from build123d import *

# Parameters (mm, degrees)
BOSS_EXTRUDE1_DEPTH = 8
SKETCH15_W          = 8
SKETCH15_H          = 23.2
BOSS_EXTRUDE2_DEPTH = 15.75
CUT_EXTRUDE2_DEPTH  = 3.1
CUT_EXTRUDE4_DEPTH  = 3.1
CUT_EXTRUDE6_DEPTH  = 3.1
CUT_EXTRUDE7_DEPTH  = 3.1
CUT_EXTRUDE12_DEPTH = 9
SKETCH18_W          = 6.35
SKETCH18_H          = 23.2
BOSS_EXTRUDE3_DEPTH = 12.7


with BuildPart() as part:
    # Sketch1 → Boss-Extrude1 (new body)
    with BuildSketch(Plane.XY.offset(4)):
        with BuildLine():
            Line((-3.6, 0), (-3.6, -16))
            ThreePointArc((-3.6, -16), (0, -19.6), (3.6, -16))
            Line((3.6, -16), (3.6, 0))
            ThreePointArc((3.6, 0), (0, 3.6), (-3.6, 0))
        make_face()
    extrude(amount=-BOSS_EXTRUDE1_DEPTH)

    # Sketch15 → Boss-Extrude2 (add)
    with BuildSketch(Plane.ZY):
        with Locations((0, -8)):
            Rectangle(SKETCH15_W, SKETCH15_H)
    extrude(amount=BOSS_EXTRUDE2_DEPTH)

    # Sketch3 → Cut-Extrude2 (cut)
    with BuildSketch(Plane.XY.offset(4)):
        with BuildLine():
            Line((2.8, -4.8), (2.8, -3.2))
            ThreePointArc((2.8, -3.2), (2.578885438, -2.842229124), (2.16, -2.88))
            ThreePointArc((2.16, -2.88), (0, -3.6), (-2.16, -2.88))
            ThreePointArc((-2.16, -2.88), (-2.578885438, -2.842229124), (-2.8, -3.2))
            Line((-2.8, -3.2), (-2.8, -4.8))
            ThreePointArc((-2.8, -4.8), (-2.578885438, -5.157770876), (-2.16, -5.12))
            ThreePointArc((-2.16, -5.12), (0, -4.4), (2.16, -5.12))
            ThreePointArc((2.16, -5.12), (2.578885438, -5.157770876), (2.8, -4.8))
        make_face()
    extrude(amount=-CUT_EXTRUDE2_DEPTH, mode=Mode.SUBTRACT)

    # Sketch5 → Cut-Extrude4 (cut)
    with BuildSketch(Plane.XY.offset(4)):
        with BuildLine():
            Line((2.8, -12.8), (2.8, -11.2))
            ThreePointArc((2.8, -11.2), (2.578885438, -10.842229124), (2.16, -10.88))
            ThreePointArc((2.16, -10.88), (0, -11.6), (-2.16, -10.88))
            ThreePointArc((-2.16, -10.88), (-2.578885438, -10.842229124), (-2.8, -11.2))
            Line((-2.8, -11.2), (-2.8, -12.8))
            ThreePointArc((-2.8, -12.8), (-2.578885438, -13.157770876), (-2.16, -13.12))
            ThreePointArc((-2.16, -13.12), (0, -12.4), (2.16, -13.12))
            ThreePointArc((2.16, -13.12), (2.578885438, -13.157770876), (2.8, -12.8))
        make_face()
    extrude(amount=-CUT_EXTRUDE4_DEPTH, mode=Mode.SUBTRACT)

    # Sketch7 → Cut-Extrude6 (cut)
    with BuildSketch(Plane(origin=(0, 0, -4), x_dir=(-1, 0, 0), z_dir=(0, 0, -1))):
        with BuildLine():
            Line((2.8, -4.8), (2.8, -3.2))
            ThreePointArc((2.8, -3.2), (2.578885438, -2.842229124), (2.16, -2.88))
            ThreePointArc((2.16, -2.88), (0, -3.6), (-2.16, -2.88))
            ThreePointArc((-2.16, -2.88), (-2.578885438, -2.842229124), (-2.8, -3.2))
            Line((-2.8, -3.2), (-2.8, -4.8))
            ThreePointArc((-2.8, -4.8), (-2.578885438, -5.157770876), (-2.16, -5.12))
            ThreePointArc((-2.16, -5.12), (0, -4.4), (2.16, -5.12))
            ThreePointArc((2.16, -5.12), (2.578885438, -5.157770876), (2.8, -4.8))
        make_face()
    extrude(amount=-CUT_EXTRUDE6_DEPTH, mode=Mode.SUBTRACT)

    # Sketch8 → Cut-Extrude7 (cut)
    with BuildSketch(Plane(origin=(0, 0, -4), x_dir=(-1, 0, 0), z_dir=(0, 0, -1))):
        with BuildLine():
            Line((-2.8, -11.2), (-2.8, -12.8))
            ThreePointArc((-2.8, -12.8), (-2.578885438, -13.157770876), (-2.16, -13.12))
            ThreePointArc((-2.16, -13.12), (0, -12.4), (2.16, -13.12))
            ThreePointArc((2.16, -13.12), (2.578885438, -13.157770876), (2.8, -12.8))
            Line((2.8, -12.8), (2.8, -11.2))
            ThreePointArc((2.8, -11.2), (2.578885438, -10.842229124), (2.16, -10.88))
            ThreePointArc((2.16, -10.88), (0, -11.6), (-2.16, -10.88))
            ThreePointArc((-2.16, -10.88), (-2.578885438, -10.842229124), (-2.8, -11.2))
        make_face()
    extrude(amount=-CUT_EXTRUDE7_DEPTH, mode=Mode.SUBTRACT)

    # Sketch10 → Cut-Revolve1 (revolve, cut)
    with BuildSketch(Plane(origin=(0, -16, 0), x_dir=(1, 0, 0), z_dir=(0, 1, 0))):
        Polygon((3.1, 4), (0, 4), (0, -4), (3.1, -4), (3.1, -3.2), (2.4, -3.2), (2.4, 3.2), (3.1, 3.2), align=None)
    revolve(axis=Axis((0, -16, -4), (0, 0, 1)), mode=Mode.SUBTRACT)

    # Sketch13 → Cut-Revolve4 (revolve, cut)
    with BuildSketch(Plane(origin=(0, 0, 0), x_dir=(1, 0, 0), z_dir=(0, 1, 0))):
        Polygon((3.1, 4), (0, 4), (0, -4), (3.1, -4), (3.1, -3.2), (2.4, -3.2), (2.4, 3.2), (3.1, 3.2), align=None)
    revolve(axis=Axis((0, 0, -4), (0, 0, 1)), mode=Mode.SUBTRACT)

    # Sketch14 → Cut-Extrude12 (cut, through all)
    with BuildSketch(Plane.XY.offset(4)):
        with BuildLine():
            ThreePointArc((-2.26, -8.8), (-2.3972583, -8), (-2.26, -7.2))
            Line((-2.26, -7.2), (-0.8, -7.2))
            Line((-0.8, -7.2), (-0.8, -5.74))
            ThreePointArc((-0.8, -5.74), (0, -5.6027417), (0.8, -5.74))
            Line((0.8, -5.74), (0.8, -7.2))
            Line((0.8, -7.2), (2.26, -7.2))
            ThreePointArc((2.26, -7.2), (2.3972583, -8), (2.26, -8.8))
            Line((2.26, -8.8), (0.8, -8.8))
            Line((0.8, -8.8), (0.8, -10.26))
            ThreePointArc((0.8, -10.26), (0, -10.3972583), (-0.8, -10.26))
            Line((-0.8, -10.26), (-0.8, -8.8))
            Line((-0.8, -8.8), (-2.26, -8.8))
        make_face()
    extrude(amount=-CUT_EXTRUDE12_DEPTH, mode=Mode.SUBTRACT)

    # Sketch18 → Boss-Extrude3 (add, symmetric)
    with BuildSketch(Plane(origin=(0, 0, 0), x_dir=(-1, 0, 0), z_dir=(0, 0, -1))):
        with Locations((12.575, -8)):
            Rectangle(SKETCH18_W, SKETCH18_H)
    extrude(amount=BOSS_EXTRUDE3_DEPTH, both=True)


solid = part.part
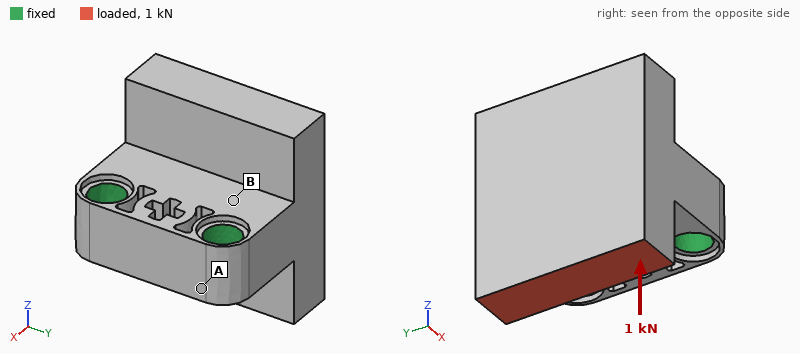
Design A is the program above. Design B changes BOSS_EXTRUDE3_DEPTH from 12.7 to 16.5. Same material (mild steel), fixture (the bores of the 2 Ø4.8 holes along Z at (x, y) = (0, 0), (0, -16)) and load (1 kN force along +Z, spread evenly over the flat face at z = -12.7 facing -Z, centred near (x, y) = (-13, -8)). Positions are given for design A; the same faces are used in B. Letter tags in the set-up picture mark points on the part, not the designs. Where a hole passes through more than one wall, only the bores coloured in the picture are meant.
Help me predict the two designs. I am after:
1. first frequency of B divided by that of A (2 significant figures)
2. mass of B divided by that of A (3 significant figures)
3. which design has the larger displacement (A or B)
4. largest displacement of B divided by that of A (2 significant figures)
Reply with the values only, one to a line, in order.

0.77
1.20
B
1.2
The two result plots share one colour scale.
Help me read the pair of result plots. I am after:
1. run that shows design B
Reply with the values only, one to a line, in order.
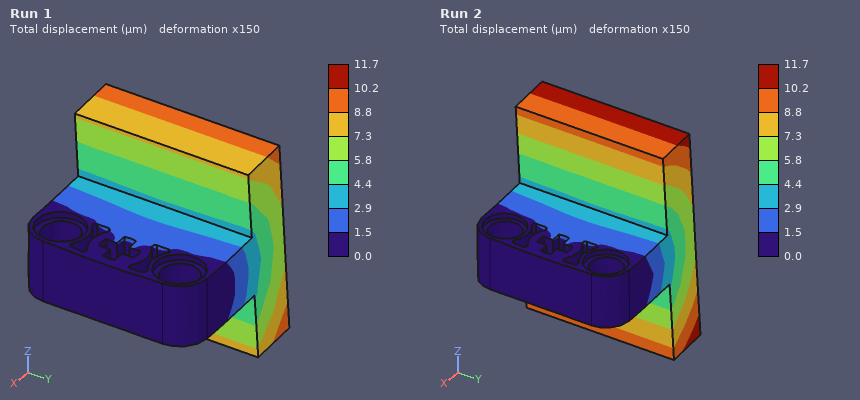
Run 2
